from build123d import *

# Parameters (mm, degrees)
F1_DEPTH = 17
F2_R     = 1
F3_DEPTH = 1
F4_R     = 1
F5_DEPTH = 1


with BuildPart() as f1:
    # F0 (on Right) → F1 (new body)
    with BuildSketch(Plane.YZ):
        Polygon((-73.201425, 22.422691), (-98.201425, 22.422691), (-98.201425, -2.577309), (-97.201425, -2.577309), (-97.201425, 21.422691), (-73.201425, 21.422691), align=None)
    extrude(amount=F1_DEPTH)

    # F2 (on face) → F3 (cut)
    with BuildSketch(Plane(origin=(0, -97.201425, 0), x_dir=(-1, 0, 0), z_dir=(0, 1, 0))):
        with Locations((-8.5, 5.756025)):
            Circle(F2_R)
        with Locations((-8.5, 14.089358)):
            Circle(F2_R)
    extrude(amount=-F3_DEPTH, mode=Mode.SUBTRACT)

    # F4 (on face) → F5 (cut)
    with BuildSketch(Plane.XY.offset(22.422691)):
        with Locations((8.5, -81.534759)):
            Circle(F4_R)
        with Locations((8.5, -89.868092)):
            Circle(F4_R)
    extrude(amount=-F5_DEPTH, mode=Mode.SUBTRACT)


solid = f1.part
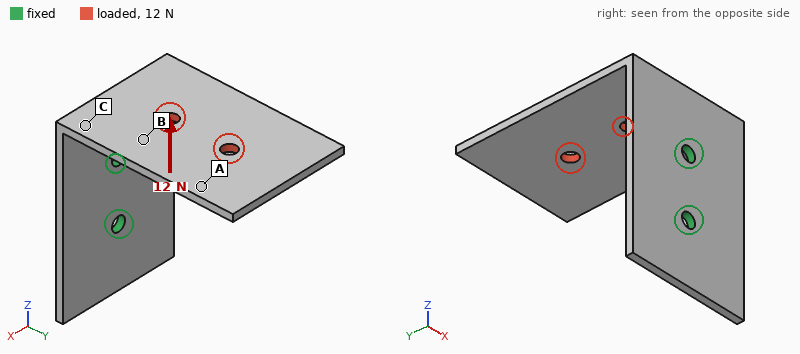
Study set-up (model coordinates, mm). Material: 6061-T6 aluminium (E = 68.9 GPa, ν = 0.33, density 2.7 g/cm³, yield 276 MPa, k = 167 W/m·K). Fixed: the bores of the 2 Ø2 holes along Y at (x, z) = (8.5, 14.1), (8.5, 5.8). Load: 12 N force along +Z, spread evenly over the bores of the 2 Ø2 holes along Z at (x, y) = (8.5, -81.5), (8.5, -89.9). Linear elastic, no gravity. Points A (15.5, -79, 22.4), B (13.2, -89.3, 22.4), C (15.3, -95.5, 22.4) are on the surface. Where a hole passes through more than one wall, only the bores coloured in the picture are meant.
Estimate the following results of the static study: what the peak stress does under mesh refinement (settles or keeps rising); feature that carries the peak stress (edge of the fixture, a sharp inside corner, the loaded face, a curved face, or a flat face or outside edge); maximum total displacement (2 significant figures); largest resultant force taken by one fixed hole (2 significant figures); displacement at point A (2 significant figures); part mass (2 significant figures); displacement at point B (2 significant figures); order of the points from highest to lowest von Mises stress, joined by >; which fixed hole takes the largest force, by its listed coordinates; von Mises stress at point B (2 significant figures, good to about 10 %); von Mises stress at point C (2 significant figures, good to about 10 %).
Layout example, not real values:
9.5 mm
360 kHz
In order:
keeps rising
edge of the fixture
0.46 mm
12 N
0.34 mm
2.2 g
0.14 mm
C > B > A
(8.5, 14.1)
18 MPa
38 MPa
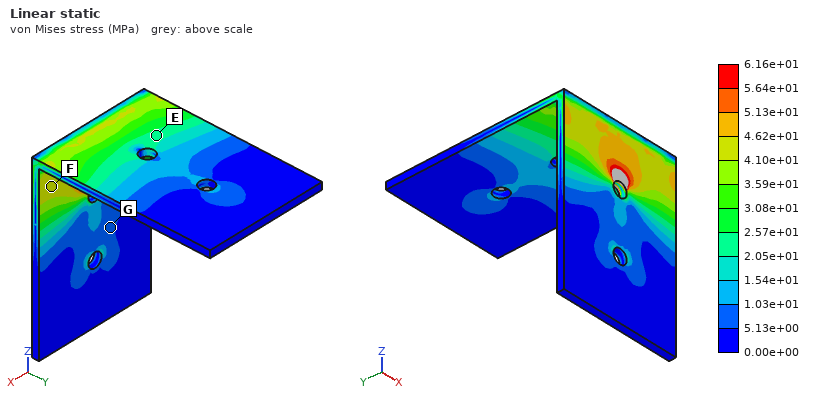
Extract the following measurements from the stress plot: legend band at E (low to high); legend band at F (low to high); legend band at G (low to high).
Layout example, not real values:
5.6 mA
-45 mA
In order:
2.05e+01 to 2.57e+01 MPa
4.10e+01 to 4.62e+01 MPa
5.13e+00 to 1.03e+01 MPa
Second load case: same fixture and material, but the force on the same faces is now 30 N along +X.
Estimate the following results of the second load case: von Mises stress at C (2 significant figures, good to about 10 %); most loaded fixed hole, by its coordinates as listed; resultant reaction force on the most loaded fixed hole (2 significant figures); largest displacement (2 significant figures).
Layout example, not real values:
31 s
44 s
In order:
40 MPa
(8.5, 14.1)
52 N
0.42 mm
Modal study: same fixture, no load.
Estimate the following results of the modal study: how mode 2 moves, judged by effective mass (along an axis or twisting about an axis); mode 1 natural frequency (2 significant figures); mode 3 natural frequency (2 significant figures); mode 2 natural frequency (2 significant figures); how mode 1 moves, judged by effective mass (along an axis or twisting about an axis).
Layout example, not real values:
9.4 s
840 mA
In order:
along X
910 Hz
4100 Hz
1500 Hz
along Z
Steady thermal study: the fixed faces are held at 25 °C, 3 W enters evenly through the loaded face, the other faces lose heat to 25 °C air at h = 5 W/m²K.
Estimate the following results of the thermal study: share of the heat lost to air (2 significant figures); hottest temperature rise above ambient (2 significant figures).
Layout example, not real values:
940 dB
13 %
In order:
3.2 %
24 K
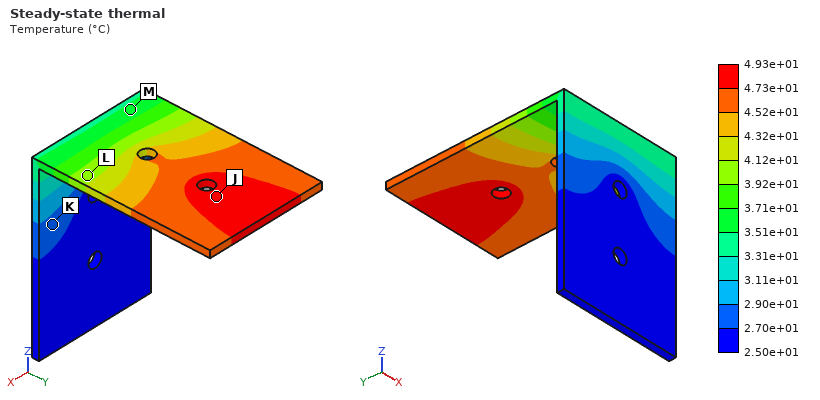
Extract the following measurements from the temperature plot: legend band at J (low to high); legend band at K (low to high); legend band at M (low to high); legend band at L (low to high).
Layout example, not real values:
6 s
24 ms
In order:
4.73e+01 to 4.93e+01 °C
2.70e+01 to 2.90e+01 °C
3.51e+01 to 3.71e+01 °C
3.92e+01 to 4.12e+01 °C
